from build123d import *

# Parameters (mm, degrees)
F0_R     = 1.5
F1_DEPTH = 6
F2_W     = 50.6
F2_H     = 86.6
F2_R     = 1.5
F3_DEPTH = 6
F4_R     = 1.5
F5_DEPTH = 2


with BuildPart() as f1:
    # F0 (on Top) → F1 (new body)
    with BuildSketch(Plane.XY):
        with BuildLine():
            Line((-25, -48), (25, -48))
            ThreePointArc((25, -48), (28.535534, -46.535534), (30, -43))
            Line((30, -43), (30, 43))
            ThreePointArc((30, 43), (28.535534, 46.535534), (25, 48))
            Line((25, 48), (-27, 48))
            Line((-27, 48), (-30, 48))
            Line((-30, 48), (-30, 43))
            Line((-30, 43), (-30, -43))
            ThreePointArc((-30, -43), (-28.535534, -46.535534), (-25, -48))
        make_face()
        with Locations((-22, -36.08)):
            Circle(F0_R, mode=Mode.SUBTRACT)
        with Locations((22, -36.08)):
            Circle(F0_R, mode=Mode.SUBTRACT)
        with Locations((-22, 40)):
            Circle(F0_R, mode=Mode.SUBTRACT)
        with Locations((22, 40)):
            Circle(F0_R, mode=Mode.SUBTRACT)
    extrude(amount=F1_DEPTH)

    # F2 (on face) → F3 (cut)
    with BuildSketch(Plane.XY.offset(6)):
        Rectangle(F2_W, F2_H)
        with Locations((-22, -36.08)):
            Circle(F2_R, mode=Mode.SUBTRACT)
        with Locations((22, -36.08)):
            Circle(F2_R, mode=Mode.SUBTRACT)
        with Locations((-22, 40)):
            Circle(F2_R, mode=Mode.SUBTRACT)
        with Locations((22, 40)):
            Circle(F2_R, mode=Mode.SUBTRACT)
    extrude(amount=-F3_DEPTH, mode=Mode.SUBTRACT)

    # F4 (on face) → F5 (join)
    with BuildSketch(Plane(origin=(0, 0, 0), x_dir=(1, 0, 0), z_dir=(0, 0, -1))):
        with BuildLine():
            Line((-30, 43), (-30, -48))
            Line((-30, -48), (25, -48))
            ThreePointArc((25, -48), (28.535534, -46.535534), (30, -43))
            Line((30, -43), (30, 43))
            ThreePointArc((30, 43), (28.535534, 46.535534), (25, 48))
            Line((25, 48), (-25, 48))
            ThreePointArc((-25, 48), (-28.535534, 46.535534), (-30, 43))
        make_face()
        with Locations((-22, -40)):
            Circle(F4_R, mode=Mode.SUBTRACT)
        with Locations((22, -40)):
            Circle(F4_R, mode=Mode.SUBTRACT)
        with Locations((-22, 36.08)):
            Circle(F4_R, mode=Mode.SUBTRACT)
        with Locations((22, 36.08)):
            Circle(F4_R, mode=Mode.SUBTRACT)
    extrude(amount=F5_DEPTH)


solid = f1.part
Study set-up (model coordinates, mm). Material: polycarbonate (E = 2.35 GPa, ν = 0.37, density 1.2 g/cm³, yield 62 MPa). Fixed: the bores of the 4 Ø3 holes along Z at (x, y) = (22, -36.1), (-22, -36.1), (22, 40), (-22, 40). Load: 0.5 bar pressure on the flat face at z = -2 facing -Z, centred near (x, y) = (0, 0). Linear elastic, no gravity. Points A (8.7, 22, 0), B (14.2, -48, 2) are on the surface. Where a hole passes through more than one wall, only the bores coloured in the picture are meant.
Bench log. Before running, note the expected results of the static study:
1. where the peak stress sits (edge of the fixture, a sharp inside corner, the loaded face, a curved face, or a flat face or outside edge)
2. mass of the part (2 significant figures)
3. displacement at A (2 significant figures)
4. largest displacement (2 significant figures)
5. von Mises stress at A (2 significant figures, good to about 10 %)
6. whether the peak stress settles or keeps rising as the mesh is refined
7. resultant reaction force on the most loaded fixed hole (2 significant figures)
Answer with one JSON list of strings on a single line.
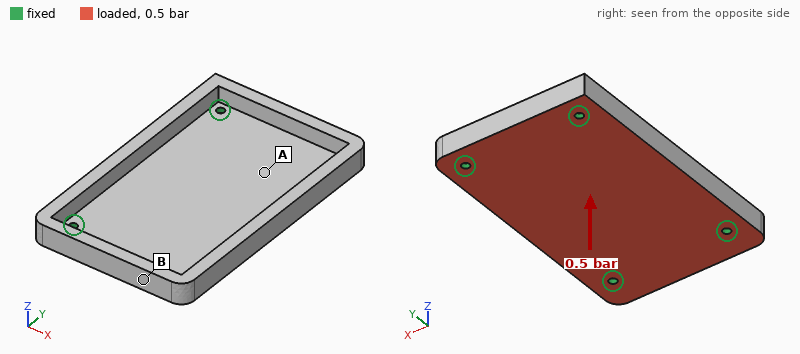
["edge of the fixture", "24 g", "0.73 mm", "1.2 mm", "5.6 MPa", "keeps rising", "93 N"]
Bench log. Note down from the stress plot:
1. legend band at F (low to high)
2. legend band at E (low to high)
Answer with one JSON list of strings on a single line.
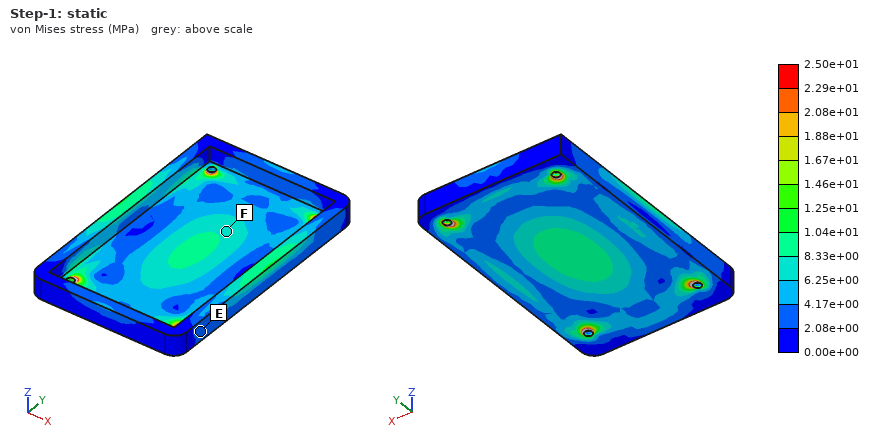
["6.25e+00 to 8.33e+00 MPa", "2.08e+00 to 4.17e+00 MPa"]
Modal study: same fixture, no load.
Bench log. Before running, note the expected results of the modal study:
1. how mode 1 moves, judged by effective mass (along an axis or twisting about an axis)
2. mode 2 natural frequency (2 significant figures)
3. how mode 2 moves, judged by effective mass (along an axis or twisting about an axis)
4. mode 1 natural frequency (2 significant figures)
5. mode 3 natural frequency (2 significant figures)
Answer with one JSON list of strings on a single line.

["along Z", "1200 Hz", "twisting about Y", "800 Hz", "1300 Hz"]
